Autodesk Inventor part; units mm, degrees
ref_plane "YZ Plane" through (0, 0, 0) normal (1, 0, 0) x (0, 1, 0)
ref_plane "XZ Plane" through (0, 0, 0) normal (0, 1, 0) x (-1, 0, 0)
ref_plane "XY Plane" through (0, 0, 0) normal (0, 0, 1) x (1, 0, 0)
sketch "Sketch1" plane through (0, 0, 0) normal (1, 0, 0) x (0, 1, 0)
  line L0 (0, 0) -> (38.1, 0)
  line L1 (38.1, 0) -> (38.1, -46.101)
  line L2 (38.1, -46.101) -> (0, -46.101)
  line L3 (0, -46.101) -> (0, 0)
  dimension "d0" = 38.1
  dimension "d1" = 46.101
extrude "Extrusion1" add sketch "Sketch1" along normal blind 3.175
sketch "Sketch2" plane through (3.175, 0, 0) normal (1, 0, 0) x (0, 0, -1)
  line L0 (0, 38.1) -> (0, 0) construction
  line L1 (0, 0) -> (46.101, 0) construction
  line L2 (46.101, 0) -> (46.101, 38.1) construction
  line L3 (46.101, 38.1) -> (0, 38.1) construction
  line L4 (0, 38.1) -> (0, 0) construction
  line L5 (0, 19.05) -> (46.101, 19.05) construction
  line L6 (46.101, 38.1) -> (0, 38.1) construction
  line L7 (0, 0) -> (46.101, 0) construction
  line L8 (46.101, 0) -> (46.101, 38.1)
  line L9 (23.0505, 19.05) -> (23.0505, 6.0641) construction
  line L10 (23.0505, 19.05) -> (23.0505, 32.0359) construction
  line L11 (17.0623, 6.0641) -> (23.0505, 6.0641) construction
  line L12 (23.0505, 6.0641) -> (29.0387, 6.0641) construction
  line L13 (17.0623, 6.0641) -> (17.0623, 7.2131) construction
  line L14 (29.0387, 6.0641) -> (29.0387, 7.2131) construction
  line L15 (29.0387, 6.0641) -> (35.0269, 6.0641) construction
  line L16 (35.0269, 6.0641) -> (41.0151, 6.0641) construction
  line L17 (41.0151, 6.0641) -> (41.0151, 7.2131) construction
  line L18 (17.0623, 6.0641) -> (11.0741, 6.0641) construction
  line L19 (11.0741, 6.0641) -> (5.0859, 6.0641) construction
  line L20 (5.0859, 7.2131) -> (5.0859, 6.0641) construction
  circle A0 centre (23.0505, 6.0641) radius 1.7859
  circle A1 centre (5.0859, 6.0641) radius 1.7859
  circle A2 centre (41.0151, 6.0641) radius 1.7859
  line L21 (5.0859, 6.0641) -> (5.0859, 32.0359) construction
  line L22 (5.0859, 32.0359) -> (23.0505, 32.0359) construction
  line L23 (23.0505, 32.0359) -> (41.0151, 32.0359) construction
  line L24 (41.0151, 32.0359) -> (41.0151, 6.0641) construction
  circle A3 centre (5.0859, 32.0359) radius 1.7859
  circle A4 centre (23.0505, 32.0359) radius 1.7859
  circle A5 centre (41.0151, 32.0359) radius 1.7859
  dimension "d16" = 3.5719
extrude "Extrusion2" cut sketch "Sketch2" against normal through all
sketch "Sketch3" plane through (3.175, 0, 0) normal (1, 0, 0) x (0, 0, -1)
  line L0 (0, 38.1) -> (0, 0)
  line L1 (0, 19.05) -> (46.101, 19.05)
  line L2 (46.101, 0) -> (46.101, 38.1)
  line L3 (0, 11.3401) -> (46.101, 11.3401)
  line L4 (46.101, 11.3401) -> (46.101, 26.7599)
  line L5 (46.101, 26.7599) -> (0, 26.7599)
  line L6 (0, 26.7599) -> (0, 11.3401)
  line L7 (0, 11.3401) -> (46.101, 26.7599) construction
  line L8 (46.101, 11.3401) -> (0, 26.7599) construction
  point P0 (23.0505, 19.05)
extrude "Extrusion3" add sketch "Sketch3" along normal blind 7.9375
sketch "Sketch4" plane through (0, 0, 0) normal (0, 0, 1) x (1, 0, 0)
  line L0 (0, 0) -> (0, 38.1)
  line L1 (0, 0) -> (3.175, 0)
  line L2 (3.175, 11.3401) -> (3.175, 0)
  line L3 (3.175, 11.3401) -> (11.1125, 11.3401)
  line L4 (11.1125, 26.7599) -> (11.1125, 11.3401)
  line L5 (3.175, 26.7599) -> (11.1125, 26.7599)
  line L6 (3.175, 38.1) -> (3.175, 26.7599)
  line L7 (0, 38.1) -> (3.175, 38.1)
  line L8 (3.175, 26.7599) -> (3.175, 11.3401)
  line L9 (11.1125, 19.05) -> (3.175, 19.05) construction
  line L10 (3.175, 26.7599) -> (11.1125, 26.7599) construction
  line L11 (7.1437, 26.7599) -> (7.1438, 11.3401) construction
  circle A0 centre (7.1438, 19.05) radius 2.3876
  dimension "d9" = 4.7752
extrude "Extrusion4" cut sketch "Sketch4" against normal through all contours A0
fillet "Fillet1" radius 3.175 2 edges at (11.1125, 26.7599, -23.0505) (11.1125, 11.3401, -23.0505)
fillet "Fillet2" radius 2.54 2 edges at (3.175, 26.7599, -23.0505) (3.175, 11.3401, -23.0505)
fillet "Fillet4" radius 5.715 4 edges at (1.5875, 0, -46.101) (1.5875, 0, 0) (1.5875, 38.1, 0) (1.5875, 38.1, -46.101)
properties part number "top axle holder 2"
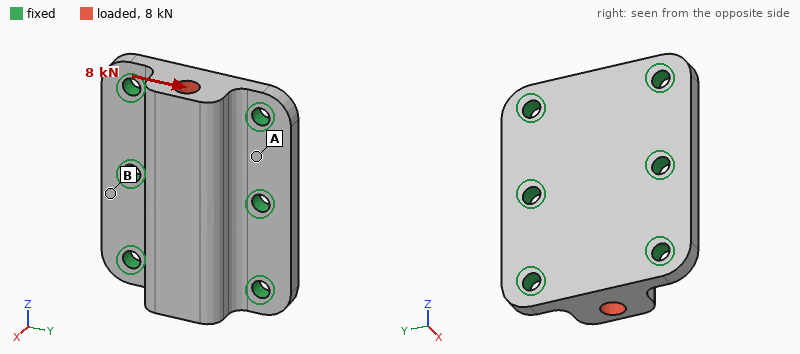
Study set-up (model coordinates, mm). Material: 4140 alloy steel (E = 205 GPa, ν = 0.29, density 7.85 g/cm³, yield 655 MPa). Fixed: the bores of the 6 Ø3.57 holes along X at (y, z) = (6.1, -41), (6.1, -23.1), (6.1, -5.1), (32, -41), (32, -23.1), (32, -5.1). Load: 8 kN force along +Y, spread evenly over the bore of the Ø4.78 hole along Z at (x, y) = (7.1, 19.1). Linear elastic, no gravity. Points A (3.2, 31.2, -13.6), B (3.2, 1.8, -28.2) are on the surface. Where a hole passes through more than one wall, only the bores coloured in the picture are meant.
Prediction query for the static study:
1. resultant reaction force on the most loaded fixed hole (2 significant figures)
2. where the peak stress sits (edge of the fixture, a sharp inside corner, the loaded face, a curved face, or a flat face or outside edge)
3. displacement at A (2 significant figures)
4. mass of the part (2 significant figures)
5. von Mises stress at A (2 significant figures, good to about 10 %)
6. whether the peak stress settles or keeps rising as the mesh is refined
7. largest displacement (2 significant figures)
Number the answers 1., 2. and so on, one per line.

1. 1.7 kN
2. edge of the fixture
3. 1.5 µm
4. 79 g
5. 21 MPa
6. keeps rising
7. 4.3 µm
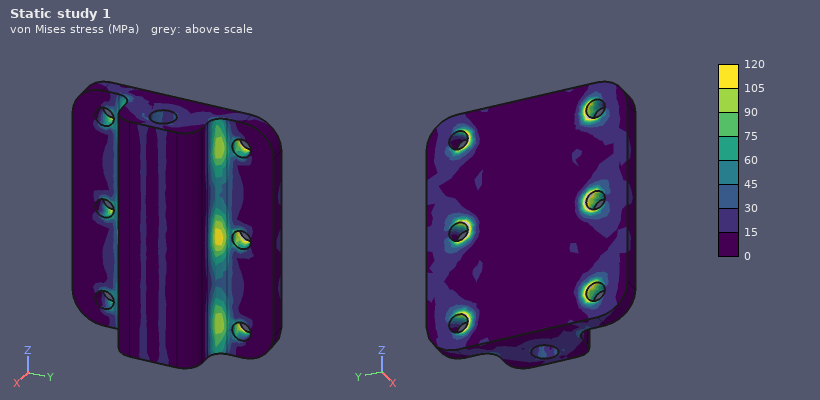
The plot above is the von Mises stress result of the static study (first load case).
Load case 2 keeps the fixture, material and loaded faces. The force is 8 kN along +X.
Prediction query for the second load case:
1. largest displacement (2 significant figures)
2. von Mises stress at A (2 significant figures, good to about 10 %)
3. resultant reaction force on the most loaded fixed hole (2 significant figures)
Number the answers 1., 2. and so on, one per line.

1. 7.2 µm
2. 25 MPa
3. 1.7 kN
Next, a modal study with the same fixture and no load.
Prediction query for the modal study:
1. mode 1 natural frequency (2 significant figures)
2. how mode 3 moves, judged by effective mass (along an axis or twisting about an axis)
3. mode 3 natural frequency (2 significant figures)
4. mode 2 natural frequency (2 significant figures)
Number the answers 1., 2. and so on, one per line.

1. 24 kHz
2. along Y
3. 37 kHz
4. 24 kHz
